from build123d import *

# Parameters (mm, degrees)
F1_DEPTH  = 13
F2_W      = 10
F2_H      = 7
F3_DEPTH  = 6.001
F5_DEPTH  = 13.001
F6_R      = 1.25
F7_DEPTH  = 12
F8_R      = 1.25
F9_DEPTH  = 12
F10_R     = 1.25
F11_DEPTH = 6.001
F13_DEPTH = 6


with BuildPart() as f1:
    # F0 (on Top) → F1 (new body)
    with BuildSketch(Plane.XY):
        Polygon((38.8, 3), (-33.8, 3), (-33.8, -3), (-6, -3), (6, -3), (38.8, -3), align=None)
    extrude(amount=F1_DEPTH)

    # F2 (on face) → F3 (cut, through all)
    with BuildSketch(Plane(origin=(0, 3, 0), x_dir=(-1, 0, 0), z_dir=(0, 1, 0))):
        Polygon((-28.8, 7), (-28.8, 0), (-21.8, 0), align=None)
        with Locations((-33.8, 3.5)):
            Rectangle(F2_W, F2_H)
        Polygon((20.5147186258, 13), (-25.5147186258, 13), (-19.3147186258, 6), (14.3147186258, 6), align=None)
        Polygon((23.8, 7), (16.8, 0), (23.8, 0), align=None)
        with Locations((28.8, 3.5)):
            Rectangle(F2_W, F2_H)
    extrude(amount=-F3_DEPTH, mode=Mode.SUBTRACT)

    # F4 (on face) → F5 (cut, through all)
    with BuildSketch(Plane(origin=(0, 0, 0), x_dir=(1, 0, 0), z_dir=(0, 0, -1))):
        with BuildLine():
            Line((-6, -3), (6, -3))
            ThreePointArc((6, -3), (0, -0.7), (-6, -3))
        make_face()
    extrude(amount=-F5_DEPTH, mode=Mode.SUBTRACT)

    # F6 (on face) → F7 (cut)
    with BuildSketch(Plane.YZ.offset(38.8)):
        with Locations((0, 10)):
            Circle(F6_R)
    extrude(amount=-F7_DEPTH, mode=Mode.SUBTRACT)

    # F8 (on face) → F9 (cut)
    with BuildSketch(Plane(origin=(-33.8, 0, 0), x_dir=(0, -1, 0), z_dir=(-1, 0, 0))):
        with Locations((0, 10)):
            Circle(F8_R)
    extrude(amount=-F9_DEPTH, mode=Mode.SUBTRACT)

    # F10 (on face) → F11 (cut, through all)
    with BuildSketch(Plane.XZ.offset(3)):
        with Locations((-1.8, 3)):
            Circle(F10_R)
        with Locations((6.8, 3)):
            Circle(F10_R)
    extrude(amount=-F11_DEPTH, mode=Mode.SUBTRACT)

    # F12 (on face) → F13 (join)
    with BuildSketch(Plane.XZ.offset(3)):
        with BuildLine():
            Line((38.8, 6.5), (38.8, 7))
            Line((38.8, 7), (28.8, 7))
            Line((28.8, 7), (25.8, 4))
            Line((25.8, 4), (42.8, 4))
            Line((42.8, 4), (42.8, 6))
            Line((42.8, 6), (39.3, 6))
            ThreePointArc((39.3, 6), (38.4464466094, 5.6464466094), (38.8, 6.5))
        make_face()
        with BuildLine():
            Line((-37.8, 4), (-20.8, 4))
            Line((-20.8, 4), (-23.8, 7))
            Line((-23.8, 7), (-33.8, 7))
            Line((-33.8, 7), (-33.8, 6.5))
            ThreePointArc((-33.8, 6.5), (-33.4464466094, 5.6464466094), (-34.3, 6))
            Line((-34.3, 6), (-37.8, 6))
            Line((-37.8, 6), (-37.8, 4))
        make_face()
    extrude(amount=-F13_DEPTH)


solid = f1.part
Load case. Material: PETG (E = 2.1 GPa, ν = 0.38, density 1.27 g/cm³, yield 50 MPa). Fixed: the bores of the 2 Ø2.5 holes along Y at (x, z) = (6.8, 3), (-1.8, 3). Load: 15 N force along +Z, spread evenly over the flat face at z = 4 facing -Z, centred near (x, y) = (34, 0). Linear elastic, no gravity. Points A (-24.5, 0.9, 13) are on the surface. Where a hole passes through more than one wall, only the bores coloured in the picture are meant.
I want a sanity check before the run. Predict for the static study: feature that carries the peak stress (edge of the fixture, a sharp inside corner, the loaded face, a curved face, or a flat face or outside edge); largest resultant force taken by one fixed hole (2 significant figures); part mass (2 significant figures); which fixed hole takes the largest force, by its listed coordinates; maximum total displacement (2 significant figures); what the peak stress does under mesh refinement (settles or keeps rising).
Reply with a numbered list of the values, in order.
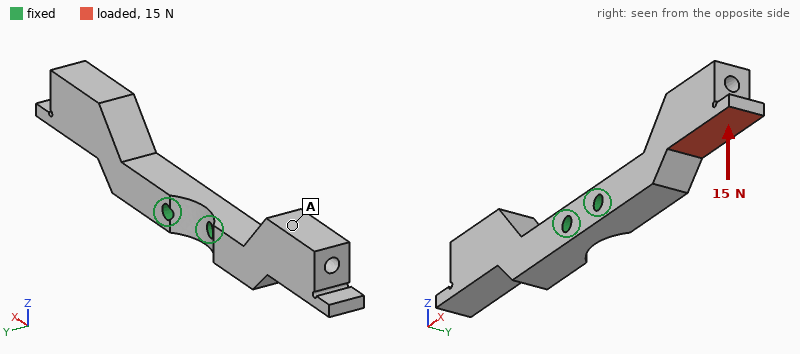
1. edge of the fixture
2. 27 N
3. 3.9 g
4. (6.8, 3)
5. 0.77 mm
6. keeps rising
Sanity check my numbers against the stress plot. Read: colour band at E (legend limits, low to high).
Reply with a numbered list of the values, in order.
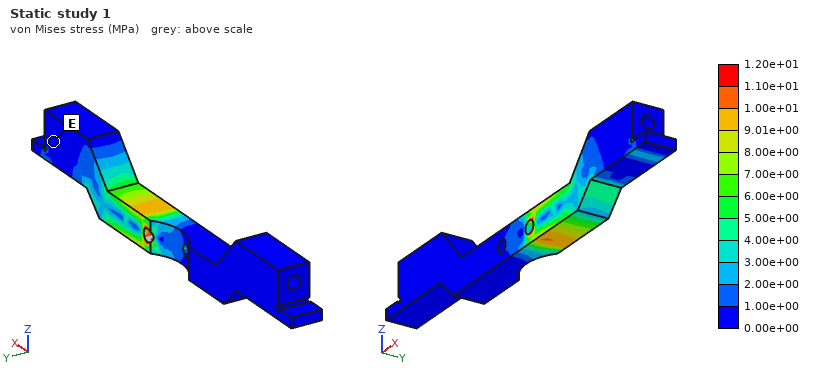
1. 0.00e+00 to 1.00e+00 MPa
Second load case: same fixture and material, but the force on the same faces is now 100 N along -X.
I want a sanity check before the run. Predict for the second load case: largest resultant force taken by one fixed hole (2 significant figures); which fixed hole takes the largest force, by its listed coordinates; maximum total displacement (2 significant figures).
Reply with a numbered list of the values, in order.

1. 96 N
2. (6.8, 3)
3. 0.10 mm
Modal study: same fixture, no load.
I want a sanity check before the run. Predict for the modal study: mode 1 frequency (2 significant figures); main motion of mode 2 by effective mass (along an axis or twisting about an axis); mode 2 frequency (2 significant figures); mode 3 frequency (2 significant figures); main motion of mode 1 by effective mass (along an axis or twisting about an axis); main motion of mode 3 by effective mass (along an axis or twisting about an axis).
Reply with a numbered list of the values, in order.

1. 760 Hz
2. along Z
3. 800 Hz
4. 870 Hz
5. along Y
6. along Z
